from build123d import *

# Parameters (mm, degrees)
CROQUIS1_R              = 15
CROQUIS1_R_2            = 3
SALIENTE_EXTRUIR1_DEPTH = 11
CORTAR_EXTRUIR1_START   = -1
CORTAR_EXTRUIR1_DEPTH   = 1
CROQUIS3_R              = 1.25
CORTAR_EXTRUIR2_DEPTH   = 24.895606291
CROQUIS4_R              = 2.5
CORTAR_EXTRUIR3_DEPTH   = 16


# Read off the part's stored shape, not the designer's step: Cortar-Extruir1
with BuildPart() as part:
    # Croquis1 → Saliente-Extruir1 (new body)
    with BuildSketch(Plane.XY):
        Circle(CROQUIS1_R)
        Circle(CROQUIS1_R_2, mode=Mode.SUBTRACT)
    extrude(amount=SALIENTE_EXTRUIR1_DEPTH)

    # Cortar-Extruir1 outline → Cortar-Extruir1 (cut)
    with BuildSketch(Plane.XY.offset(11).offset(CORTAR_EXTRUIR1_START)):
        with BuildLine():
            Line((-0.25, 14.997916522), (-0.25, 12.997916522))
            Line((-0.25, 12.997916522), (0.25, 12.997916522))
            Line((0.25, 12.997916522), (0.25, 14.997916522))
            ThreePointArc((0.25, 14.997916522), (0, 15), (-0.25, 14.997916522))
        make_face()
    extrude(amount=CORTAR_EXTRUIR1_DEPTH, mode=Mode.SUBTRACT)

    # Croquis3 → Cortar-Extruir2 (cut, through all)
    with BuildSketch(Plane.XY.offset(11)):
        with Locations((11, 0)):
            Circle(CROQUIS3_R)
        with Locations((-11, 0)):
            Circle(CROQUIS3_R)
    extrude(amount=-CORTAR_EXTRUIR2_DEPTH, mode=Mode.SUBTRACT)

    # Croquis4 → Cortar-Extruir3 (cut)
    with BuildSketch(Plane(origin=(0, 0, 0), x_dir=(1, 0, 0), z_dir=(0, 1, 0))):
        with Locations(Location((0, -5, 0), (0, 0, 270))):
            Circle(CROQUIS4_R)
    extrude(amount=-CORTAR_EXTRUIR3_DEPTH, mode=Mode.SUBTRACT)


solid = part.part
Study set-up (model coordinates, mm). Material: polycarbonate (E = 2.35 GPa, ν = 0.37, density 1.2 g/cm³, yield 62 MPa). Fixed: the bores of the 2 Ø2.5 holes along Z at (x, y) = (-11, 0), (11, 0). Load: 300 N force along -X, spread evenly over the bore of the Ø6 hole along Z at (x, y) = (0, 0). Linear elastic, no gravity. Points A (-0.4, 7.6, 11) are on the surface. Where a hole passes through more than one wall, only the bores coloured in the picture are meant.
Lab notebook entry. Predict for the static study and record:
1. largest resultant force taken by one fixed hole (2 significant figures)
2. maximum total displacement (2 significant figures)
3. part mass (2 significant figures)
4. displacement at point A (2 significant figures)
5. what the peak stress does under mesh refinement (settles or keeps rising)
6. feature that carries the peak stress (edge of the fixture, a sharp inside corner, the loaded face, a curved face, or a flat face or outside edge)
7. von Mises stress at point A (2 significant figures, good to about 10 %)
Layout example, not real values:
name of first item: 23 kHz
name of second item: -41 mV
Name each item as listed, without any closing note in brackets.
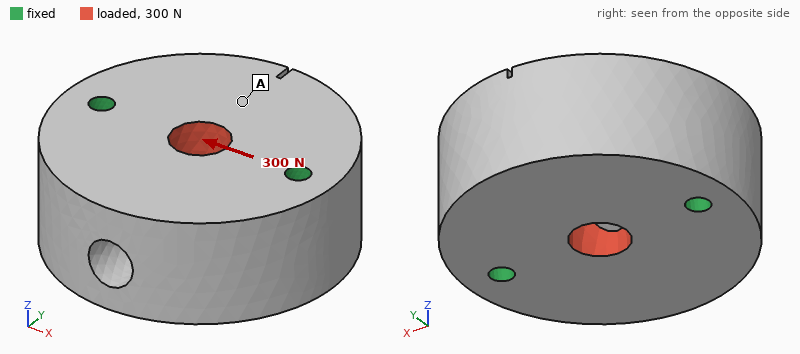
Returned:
largest resultant force taken by one fixed hole: 150 N
maximum total displacement: 7.6 µm
part mass: 8.5 g
displacement at point A: 4.1 µm
what the peak stress does under mesh refinement: keeps rising
feature that carries the peak stress: edge of the fixture
von Mises stress at point A: 0.42 MPa
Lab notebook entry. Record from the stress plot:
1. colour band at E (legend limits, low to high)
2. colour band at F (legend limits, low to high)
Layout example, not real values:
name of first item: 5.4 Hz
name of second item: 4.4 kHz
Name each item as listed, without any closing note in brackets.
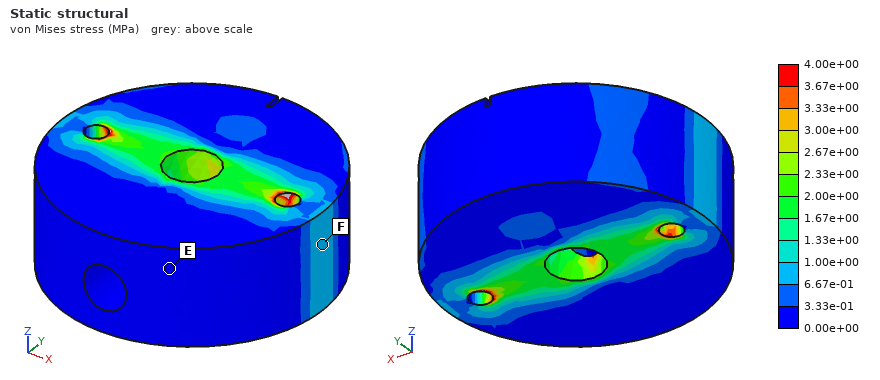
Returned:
colour band at E: 0.00e+00 to 3.33e-01 MPa
colour band at F: 6.67e-01 to 1.00e+00 MPa
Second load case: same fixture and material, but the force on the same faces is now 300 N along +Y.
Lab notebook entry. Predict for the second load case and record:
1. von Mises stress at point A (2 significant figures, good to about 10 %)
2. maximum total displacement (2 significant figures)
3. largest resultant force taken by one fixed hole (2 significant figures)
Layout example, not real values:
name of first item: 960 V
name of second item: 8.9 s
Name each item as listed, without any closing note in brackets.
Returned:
von Mises stress at point A: 1.1 MPa
maximum total displacement: 11 µm
largest resultant force taken by one fixed hole: 150 N
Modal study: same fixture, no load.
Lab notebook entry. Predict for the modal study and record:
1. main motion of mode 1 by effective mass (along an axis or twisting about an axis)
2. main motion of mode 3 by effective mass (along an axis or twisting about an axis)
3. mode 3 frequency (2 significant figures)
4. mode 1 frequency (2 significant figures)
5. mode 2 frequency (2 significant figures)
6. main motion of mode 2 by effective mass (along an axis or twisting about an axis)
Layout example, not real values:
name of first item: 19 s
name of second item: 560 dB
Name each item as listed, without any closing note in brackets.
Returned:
main motion of mode 1 by effective mass: twisting about X
main motion of mode 3 by effective mass: twisting about Z
mode 3 frequency: 13 kHz
mode 1 frequency: 7000 Hz
mode 2 frequency: 8700 Hz
main motion of mode 2 by effective mass: along Z
